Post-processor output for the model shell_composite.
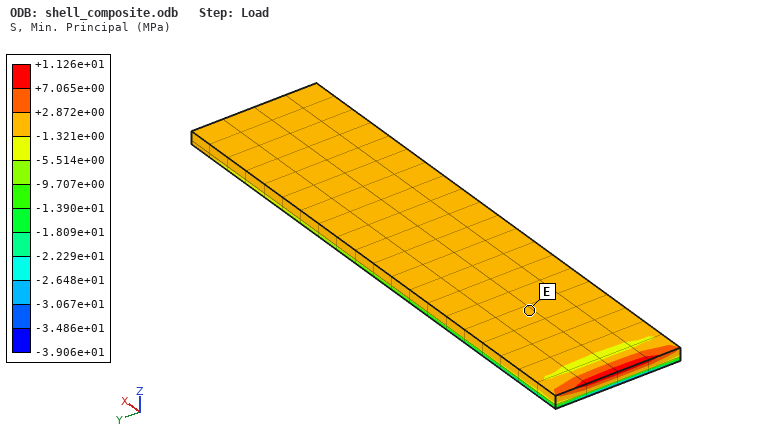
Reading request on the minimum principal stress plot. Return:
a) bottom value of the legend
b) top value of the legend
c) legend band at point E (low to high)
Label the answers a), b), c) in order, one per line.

a) -3.906e+01 MPa
b) +1.126e+01 MPa
c) -1.321e+00 to +2.872e+00 MPa
